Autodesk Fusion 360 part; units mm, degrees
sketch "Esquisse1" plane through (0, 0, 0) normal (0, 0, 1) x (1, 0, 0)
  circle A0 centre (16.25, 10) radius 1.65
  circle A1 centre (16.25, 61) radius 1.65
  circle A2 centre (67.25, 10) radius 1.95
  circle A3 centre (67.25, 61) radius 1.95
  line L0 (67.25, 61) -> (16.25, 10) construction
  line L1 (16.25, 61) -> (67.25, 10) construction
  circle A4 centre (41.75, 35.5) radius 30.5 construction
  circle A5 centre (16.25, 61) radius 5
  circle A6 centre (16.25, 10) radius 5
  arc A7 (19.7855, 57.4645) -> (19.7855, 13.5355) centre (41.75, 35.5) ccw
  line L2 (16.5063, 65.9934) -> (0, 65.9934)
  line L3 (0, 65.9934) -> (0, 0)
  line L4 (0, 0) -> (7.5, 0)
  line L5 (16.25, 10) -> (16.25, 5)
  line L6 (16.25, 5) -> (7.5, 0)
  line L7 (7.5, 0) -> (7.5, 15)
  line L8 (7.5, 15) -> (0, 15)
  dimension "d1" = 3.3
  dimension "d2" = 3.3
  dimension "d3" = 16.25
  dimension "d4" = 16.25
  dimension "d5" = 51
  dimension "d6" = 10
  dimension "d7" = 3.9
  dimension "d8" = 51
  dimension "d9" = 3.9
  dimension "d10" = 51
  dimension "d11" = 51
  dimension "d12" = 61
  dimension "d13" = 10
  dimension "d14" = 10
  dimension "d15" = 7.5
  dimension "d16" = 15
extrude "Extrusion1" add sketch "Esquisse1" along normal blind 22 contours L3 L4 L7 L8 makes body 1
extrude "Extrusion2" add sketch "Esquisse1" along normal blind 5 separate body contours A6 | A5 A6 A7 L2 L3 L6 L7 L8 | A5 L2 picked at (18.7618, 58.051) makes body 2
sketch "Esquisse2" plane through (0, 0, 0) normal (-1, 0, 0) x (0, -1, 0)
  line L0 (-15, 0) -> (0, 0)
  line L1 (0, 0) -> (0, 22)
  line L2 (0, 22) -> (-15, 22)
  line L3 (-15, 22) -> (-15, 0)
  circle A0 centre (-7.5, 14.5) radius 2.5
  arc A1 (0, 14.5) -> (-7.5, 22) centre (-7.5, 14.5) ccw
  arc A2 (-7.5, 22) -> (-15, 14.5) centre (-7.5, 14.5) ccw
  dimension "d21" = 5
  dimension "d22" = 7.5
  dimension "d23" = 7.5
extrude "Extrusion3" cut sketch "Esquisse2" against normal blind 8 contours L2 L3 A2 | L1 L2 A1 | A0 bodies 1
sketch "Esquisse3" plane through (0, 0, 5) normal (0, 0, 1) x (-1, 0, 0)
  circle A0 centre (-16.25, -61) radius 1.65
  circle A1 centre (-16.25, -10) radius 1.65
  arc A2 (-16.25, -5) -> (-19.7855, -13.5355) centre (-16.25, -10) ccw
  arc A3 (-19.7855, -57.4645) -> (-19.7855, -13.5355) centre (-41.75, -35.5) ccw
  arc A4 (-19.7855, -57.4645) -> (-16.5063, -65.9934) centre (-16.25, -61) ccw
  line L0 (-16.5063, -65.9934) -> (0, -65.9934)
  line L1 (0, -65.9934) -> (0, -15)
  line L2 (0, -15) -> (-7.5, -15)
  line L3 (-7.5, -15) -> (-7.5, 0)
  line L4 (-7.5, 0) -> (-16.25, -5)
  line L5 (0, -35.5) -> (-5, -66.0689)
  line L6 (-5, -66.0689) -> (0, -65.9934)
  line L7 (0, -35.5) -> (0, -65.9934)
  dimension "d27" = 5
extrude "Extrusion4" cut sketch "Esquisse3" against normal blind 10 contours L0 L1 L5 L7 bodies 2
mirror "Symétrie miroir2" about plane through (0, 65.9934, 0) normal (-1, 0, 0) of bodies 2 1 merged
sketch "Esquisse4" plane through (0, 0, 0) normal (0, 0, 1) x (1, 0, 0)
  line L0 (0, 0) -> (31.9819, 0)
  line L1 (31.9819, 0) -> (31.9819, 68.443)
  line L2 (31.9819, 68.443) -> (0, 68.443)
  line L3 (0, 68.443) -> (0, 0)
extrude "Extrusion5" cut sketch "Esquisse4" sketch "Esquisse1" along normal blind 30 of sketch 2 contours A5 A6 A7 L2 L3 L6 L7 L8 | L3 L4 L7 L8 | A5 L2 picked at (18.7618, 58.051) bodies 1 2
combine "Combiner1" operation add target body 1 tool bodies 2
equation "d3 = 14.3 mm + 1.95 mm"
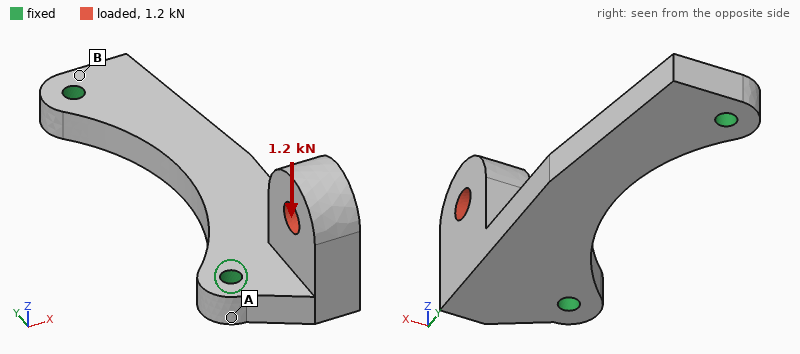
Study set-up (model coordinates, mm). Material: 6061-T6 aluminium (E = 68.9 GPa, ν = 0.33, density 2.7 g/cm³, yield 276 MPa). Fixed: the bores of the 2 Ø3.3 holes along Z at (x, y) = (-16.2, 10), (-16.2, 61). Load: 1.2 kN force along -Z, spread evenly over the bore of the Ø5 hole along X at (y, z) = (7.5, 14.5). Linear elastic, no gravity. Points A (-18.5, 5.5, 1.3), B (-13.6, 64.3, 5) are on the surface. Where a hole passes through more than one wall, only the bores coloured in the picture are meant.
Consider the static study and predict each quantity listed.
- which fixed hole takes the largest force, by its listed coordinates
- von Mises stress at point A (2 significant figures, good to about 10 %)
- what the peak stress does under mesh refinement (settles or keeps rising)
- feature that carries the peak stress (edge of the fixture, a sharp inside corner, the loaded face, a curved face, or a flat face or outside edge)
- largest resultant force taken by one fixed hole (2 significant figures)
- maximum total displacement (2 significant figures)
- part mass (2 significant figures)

(-16.2, 10)
56 MPa
keeps rising
edge of the fixture
1.2 kN
0.20 mm
17 g
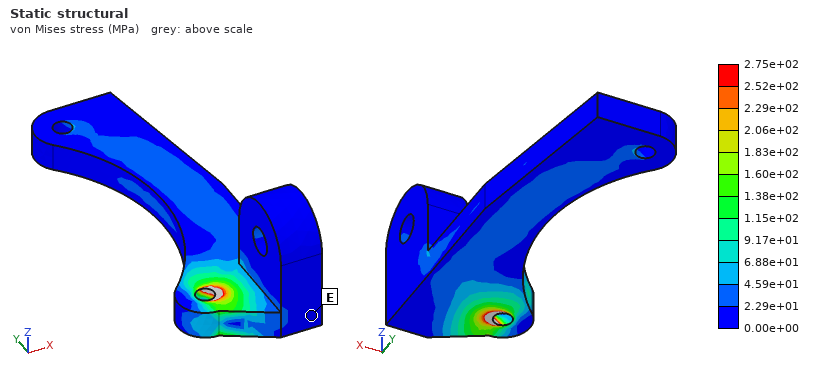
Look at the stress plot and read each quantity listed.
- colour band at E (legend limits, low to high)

0.00e+00 to 2.29e+01 MPa
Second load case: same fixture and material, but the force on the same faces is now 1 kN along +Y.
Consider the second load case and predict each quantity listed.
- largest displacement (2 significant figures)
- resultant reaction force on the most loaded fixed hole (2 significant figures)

0.14 mm
570 N
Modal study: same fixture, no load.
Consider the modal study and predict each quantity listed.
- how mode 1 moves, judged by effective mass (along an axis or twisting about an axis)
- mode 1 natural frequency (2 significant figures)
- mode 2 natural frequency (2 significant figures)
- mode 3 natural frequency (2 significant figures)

along Z
5000 Hz
6600 Hz
11 kHz
